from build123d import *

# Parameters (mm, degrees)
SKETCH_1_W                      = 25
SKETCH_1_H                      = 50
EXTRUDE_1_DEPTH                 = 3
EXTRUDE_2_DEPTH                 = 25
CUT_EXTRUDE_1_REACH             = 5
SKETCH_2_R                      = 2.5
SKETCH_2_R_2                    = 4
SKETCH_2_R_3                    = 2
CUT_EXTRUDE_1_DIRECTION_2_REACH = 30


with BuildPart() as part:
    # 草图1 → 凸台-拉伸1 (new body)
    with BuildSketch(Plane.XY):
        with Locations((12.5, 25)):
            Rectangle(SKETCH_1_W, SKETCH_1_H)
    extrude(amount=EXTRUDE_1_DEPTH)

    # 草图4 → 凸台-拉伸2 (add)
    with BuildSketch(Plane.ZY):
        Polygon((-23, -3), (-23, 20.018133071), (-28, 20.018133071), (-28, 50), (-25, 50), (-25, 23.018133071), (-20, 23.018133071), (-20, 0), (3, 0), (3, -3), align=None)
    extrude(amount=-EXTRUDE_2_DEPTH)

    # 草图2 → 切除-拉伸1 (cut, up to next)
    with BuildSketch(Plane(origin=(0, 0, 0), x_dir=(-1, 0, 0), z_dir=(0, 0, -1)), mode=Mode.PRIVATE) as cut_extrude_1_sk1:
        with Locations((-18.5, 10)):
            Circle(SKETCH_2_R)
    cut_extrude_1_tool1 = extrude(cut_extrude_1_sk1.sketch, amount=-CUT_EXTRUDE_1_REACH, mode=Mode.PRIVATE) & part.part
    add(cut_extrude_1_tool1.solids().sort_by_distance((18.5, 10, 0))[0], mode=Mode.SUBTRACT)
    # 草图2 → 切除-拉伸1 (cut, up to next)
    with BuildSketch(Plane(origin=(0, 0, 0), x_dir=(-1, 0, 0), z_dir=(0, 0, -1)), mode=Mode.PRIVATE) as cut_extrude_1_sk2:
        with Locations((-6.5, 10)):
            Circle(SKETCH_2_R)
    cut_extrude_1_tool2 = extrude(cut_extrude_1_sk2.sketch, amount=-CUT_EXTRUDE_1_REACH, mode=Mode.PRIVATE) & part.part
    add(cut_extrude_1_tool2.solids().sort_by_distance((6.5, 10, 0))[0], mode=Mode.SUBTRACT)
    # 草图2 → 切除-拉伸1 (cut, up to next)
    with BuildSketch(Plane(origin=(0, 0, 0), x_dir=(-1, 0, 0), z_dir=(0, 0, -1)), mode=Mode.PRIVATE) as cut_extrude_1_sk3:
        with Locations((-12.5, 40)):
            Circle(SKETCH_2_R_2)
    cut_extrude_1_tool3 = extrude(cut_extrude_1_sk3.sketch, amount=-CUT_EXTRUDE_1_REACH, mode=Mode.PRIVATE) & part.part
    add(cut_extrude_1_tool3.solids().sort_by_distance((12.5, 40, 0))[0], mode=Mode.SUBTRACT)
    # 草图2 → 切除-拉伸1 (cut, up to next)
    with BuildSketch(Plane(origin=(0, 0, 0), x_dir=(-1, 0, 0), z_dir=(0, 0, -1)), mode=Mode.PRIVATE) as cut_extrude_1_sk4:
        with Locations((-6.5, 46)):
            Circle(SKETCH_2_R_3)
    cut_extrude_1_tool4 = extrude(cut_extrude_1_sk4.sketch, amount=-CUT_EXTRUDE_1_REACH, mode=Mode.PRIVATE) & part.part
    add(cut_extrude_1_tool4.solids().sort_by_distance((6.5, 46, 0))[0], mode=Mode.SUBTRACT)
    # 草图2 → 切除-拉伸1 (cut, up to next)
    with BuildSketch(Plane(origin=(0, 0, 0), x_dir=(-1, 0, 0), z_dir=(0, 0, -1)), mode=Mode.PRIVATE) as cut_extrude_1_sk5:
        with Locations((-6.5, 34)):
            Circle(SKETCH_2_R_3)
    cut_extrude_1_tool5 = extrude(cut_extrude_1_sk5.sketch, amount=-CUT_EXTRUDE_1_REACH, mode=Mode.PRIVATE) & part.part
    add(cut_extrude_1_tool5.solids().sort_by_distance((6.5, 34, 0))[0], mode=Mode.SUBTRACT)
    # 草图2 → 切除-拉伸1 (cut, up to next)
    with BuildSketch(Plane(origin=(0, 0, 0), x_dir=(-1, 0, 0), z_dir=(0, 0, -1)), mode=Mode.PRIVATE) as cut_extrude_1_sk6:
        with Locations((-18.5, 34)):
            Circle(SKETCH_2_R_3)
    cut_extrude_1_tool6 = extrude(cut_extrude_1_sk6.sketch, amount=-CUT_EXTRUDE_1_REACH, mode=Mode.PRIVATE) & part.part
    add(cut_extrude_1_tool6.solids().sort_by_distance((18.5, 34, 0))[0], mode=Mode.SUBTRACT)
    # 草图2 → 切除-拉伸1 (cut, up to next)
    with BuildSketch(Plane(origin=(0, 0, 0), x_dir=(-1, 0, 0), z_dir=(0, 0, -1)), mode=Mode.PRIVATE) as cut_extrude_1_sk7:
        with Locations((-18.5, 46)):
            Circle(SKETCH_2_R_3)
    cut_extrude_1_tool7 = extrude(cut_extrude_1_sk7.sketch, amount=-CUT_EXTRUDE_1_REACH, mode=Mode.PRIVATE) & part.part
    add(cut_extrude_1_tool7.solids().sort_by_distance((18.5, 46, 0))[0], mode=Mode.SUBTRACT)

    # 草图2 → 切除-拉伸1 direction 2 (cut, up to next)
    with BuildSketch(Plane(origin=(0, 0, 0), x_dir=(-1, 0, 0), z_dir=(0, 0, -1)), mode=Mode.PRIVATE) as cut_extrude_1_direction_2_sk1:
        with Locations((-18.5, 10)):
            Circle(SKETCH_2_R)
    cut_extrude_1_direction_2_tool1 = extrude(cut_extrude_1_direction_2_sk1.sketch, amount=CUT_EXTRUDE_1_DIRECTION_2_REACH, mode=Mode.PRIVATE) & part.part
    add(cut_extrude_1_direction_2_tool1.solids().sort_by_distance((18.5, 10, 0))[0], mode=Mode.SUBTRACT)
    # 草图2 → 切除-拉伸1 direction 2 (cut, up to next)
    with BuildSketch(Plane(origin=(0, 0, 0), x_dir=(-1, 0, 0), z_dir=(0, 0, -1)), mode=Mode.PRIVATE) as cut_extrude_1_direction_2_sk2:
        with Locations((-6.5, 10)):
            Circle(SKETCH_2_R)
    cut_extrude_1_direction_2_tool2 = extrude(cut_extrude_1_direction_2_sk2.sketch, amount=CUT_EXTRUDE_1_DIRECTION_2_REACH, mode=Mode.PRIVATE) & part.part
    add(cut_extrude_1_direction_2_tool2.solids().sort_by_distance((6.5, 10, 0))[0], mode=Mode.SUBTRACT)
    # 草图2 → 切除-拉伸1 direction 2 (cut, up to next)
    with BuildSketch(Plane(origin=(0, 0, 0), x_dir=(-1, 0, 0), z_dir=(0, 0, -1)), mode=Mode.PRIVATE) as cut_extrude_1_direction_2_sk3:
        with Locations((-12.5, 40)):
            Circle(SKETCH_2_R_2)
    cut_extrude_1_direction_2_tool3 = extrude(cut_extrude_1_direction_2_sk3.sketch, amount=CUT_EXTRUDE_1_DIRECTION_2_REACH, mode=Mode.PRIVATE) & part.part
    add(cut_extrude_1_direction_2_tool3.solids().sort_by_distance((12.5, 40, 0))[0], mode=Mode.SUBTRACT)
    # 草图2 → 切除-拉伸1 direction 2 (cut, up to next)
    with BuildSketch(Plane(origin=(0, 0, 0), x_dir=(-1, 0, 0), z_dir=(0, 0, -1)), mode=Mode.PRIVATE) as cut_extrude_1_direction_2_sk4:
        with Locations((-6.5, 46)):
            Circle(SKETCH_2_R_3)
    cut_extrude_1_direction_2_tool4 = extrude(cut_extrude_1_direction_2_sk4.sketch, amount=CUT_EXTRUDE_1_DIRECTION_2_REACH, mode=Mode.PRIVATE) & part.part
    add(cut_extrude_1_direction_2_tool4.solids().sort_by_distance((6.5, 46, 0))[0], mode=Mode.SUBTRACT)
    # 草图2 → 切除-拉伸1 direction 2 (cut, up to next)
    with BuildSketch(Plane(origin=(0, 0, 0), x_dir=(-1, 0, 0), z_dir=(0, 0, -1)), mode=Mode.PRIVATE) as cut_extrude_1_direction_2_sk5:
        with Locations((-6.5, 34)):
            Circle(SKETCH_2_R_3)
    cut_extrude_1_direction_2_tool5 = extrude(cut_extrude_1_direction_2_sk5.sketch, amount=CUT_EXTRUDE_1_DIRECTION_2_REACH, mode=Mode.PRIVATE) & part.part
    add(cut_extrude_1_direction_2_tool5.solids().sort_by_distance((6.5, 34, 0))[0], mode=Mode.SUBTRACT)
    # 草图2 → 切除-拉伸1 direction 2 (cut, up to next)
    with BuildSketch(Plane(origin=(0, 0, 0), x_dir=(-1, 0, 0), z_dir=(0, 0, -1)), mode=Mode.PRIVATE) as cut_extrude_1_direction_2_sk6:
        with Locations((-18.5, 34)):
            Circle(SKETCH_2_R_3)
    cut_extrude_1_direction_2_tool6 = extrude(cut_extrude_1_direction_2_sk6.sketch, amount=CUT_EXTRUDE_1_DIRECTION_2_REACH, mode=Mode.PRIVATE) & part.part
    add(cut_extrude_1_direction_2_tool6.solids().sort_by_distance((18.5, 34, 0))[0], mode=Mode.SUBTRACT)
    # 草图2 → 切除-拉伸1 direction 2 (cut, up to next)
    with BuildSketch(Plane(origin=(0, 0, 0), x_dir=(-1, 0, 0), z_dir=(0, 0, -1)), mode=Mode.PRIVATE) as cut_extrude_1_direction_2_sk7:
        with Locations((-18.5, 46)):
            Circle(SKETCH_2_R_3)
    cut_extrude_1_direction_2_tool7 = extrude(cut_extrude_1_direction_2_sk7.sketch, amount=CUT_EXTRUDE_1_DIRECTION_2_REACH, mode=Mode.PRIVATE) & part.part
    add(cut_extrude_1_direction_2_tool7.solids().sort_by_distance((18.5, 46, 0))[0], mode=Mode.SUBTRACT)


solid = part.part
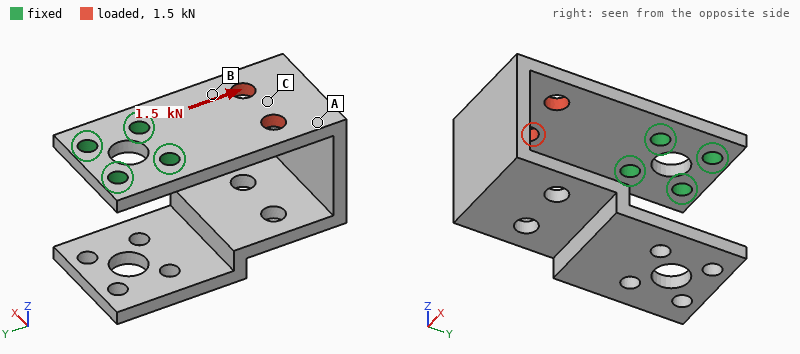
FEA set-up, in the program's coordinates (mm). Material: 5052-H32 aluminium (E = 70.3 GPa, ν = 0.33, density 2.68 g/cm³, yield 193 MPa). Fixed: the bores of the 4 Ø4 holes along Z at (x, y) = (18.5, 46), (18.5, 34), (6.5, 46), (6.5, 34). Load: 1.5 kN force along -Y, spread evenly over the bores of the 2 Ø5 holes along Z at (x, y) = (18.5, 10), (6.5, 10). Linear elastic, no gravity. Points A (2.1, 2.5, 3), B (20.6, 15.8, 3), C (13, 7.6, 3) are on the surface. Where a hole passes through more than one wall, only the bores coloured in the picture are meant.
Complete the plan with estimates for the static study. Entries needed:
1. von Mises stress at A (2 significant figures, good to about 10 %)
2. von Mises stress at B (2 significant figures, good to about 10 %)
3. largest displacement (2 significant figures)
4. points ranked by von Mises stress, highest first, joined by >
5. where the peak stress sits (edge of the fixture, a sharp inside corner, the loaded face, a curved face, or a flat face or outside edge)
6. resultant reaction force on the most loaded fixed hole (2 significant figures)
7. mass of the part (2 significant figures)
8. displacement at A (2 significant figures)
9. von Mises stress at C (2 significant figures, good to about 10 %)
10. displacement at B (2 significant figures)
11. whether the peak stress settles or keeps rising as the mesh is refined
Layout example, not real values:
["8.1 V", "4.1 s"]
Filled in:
["4.8 MPa", "21 MPa", "8.7 µm", "B > C > A", "edge of the fixture", "700 N", "24 g", "7.5 µm", "11 MPa", "5.4 µm", "keeps rising"]
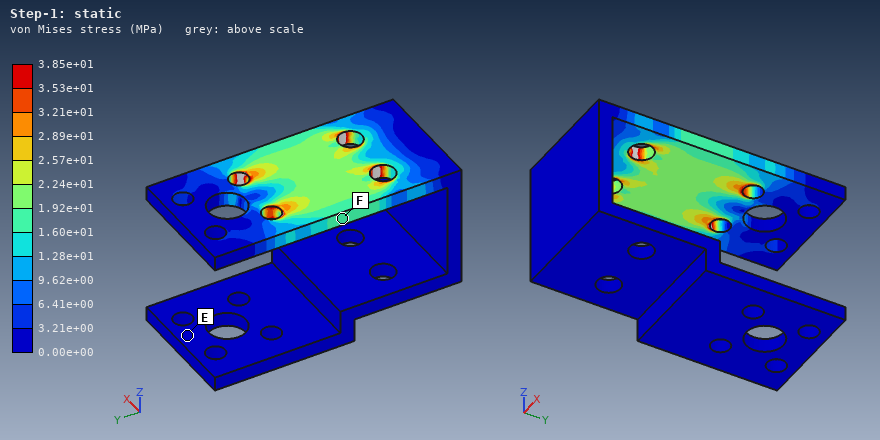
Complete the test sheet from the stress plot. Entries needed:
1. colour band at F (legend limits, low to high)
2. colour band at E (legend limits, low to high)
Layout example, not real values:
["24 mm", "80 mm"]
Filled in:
["1.60e+01 to 1.92e+01 MPa", "0.00e+00 to 3.21e+00 MPa"]
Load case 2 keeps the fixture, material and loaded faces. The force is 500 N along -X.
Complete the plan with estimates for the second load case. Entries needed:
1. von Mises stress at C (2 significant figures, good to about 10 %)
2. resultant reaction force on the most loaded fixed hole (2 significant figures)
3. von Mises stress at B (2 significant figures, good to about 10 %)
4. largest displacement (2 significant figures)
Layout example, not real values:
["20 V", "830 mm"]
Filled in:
["5.6 MPa", "690 N", "10 MPa", "28 µm"]
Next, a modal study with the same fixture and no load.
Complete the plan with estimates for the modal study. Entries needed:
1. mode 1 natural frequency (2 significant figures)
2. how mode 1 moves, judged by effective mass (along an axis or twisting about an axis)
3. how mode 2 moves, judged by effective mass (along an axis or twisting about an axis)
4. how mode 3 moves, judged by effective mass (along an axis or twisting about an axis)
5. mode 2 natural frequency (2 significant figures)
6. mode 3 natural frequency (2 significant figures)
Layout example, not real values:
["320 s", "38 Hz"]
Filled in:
["400 Hz", "along Y", "along X", "along Z", "590 Hz", "770 Hz"]
